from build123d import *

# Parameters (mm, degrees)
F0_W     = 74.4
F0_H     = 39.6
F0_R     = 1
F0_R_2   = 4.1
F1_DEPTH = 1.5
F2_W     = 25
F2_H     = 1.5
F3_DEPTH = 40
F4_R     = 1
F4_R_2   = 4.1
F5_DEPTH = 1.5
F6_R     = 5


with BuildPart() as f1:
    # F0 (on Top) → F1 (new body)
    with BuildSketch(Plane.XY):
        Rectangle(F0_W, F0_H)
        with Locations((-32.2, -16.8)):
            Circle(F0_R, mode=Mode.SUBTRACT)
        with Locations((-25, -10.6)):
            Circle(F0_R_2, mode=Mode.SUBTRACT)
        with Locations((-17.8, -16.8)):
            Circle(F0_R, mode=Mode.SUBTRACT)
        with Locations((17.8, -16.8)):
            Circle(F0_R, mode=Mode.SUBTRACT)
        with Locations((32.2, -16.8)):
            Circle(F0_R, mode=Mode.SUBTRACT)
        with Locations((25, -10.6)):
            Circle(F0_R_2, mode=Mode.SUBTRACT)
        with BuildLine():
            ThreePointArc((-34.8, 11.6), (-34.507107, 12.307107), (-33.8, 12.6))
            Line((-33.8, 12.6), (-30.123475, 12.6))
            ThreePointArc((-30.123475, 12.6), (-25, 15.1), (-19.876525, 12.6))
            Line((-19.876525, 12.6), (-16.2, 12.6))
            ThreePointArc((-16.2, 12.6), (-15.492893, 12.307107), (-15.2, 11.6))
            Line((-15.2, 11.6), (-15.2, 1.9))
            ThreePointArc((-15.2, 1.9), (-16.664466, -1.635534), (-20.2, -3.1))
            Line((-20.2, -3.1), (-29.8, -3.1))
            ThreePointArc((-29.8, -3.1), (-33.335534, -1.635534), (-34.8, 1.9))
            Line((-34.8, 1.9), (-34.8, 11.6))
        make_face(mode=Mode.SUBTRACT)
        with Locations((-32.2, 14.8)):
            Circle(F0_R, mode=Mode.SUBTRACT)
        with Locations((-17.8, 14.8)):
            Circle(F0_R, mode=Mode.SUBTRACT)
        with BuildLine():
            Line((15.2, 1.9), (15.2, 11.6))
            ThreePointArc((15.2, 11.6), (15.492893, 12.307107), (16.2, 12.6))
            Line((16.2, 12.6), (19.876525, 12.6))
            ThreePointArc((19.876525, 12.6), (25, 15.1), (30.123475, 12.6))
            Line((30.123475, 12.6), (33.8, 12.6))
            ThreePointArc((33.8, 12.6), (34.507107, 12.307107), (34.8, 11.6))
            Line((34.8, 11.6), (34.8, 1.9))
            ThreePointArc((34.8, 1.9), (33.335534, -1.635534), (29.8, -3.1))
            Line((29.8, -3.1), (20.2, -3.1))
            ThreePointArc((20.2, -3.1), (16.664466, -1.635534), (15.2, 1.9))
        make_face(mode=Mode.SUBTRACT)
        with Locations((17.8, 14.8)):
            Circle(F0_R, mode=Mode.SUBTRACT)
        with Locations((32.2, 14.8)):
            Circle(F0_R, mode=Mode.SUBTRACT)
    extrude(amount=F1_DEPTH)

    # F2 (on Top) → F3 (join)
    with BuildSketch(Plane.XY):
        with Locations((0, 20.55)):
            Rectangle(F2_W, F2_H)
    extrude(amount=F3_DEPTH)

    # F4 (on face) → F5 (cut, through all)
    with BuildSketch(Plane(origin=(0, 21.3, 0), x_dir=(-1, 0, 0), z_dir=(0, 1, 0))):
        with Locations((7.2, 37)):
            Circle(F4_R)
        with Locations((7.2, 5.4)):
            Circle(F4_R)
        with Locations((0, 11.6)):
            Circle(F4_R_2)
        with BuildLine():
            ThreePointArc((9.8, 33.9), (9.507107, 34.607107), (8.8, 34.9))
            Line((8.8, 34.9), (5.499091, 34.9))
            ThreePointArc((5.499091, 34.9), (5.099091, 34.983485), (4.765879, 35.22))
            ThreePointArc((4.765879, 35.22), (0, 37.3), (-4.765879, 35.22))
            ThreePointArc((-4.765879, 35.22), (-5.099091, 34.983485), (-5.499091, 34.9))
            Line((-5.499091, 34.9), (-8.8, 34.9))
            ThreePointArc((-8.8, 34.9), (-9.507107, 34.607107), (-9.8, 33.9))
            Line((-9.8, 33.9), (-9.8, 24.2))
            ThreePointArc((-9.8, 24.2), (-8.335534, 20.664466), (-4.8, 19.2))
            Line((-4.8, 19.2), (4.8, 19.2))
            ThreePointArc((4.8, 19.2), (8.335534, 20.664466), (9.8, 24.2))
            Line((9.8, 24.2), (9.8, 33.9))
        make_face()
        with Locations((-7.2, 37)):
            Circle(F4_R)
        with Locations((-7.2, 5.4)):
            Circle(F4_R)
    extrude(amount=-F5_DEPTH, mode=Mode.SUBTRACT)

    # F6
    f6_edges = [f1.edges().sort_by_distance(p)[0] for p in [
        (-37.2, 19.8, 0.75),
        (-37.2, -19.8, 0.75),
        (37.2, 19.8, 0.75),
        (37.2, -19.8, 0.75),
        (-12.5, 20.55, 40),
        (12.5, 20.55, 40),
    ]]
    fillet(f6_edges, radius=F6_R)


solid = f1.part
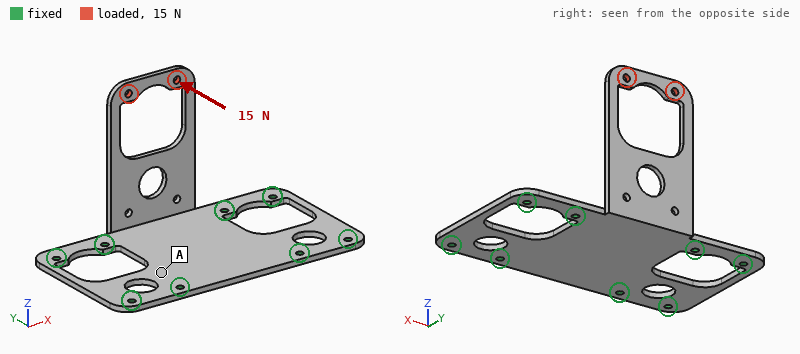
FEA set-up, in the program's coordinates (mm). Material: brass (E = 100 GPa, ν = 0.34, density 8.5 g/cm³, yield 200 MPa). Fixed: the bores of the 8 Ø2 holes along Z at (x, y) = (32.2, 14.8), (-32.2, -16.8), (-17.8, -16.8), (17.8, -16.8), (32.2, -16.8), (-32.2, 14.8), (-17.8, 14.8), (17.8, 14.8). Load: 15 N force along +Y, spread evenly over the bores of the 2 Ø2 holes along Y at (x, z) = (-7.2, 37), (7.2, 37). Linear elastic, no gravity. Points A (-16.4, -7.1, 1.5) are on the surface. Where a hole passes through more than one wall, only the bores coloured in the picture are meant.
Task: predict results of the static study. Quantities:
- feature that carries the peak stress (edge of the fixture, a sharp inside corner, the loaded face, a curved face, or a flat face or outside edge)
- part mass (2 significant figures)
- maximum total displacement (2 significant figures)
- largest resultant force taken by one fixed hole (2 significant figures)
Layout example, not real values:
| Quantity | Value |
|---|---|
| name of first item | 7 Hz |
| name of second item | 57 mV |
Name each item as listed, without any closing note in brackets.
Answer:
| Quantity | Value |
|---|---|
| feature that carries the peak stress | a curved face |
| part mass | 35 g |
| maximum total displacement | 0.84 mm |
| largest resultant force taken by one fixed hole | 9.5 N |
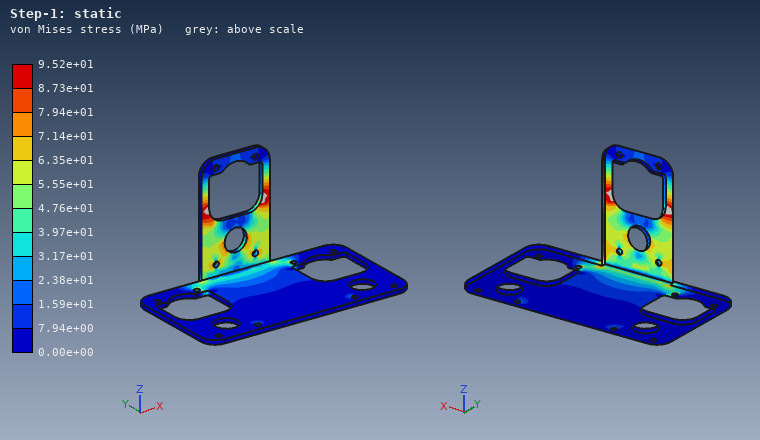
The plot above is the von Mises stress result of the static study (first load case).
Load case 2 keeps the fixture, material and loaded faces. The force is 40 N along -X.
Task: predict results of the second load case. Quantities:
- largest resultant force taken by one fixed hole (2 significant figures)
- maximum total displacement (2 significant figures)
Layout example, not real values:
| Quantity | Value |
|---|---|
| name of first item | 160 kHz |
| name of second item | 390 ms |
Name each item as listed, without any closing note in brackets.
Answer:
| Quantity | Value |
|---|---|
| largest resultant force taken by one fixed hole | 57 N |
| maximum total displacement | 0.10 mm |
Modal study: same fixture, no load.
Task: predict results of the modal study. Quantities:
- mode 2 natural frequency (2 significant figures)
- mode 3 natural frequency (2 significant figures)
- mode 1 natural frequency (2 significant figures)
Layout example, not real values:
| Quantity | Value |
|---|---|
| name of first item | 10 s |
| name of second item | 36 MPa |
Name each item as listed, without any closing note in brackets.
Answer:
| Quantity | Value |
|---|---|
| mode 2 natural frequency | 1600 Hz |
| mode 3 natural frequency | 2200 Hz |
| mode 1 natural frequency | 530 Hz |
